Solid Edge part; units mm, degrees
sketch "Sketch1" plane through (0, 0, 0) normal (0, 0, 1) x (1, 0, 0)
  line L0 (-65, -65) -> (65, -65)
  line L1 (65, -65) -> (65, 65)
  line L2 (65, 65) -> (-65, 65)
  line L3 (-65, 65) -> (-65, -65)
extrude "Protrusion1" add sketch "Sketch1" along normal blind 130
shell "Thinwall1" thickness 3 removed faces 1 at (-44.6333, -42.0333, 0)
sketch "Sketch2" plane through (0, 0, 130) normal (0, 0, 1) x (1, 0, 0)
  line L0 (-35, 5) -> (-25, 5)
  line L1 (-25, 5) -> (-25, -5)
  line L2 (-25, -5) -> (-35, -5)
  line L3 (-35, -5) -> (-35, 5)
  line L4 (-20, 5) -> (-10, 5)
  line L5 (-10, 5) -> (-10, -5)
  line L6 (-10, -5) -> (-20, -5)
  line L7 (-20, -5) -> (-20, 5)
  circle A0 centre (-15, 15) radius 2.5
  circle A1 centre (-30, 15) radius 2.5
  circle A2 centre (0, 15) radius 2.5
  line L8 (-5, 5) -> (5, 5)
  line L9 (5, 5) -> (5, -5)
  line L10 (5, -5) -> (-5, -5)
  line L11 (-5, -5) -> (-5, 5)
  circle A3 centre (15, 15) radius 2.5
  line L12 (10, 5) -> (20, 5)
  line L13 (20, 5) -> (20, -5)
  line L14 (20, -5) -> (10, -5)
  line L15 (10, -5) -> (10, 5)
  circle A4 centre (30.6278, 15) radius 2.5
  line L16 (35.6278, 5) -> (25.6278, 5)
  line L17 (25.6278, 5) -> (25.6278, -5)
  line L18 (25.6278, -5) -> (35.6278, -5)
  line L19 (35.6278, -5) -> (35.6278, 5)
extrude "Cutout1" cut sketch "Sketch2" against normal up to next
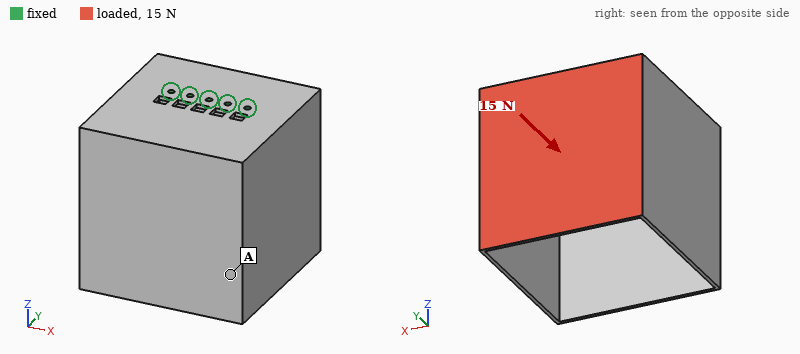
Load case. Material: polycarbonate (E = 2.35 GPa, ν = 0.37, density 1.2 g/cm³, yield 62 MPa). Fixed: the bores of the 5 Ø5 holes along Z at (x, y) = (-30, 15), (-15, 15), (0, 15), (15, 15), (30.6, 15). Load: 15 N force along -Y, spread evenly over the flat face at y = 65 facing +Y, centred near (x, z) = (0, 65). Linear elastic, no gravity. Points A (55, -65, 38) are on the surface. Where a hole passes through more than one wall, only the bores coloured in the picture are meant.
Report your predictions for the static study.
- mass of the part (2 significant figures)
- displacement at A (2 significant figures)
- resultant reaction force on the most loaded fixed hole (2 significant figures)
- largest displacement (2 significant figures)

290 g
1.9 mm
5.9 N
2.3 mm
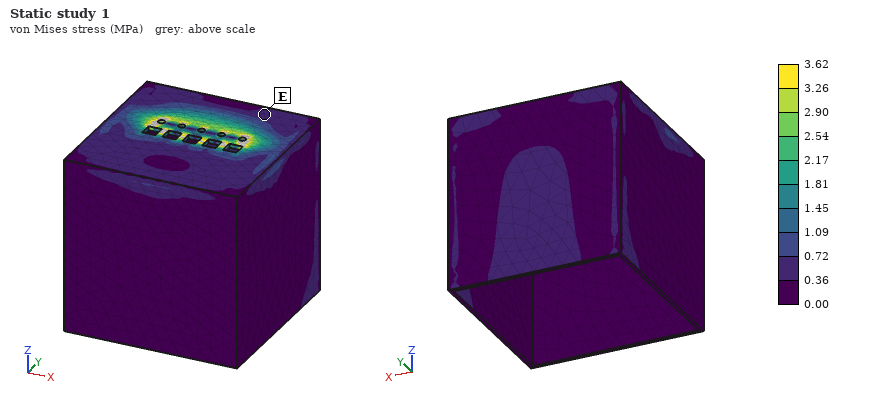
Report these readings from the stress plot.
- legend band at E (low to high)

0.36 to 0.72 MPa
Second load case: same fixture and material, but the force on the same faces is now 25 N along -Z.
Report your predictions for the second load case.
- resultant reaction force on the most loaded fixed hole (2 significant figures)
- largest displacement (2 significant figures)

9.5 N
2.6 mm
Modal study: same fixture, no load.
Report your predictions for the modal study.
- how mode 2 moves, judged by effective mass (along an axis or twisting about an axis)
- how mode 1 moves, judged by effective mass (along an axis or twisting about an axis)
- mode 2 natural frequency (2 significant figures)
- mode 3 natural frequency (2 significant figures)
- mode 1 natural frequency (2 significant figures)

along X
along Y
59 Hz
85 Hz
28 Hz
